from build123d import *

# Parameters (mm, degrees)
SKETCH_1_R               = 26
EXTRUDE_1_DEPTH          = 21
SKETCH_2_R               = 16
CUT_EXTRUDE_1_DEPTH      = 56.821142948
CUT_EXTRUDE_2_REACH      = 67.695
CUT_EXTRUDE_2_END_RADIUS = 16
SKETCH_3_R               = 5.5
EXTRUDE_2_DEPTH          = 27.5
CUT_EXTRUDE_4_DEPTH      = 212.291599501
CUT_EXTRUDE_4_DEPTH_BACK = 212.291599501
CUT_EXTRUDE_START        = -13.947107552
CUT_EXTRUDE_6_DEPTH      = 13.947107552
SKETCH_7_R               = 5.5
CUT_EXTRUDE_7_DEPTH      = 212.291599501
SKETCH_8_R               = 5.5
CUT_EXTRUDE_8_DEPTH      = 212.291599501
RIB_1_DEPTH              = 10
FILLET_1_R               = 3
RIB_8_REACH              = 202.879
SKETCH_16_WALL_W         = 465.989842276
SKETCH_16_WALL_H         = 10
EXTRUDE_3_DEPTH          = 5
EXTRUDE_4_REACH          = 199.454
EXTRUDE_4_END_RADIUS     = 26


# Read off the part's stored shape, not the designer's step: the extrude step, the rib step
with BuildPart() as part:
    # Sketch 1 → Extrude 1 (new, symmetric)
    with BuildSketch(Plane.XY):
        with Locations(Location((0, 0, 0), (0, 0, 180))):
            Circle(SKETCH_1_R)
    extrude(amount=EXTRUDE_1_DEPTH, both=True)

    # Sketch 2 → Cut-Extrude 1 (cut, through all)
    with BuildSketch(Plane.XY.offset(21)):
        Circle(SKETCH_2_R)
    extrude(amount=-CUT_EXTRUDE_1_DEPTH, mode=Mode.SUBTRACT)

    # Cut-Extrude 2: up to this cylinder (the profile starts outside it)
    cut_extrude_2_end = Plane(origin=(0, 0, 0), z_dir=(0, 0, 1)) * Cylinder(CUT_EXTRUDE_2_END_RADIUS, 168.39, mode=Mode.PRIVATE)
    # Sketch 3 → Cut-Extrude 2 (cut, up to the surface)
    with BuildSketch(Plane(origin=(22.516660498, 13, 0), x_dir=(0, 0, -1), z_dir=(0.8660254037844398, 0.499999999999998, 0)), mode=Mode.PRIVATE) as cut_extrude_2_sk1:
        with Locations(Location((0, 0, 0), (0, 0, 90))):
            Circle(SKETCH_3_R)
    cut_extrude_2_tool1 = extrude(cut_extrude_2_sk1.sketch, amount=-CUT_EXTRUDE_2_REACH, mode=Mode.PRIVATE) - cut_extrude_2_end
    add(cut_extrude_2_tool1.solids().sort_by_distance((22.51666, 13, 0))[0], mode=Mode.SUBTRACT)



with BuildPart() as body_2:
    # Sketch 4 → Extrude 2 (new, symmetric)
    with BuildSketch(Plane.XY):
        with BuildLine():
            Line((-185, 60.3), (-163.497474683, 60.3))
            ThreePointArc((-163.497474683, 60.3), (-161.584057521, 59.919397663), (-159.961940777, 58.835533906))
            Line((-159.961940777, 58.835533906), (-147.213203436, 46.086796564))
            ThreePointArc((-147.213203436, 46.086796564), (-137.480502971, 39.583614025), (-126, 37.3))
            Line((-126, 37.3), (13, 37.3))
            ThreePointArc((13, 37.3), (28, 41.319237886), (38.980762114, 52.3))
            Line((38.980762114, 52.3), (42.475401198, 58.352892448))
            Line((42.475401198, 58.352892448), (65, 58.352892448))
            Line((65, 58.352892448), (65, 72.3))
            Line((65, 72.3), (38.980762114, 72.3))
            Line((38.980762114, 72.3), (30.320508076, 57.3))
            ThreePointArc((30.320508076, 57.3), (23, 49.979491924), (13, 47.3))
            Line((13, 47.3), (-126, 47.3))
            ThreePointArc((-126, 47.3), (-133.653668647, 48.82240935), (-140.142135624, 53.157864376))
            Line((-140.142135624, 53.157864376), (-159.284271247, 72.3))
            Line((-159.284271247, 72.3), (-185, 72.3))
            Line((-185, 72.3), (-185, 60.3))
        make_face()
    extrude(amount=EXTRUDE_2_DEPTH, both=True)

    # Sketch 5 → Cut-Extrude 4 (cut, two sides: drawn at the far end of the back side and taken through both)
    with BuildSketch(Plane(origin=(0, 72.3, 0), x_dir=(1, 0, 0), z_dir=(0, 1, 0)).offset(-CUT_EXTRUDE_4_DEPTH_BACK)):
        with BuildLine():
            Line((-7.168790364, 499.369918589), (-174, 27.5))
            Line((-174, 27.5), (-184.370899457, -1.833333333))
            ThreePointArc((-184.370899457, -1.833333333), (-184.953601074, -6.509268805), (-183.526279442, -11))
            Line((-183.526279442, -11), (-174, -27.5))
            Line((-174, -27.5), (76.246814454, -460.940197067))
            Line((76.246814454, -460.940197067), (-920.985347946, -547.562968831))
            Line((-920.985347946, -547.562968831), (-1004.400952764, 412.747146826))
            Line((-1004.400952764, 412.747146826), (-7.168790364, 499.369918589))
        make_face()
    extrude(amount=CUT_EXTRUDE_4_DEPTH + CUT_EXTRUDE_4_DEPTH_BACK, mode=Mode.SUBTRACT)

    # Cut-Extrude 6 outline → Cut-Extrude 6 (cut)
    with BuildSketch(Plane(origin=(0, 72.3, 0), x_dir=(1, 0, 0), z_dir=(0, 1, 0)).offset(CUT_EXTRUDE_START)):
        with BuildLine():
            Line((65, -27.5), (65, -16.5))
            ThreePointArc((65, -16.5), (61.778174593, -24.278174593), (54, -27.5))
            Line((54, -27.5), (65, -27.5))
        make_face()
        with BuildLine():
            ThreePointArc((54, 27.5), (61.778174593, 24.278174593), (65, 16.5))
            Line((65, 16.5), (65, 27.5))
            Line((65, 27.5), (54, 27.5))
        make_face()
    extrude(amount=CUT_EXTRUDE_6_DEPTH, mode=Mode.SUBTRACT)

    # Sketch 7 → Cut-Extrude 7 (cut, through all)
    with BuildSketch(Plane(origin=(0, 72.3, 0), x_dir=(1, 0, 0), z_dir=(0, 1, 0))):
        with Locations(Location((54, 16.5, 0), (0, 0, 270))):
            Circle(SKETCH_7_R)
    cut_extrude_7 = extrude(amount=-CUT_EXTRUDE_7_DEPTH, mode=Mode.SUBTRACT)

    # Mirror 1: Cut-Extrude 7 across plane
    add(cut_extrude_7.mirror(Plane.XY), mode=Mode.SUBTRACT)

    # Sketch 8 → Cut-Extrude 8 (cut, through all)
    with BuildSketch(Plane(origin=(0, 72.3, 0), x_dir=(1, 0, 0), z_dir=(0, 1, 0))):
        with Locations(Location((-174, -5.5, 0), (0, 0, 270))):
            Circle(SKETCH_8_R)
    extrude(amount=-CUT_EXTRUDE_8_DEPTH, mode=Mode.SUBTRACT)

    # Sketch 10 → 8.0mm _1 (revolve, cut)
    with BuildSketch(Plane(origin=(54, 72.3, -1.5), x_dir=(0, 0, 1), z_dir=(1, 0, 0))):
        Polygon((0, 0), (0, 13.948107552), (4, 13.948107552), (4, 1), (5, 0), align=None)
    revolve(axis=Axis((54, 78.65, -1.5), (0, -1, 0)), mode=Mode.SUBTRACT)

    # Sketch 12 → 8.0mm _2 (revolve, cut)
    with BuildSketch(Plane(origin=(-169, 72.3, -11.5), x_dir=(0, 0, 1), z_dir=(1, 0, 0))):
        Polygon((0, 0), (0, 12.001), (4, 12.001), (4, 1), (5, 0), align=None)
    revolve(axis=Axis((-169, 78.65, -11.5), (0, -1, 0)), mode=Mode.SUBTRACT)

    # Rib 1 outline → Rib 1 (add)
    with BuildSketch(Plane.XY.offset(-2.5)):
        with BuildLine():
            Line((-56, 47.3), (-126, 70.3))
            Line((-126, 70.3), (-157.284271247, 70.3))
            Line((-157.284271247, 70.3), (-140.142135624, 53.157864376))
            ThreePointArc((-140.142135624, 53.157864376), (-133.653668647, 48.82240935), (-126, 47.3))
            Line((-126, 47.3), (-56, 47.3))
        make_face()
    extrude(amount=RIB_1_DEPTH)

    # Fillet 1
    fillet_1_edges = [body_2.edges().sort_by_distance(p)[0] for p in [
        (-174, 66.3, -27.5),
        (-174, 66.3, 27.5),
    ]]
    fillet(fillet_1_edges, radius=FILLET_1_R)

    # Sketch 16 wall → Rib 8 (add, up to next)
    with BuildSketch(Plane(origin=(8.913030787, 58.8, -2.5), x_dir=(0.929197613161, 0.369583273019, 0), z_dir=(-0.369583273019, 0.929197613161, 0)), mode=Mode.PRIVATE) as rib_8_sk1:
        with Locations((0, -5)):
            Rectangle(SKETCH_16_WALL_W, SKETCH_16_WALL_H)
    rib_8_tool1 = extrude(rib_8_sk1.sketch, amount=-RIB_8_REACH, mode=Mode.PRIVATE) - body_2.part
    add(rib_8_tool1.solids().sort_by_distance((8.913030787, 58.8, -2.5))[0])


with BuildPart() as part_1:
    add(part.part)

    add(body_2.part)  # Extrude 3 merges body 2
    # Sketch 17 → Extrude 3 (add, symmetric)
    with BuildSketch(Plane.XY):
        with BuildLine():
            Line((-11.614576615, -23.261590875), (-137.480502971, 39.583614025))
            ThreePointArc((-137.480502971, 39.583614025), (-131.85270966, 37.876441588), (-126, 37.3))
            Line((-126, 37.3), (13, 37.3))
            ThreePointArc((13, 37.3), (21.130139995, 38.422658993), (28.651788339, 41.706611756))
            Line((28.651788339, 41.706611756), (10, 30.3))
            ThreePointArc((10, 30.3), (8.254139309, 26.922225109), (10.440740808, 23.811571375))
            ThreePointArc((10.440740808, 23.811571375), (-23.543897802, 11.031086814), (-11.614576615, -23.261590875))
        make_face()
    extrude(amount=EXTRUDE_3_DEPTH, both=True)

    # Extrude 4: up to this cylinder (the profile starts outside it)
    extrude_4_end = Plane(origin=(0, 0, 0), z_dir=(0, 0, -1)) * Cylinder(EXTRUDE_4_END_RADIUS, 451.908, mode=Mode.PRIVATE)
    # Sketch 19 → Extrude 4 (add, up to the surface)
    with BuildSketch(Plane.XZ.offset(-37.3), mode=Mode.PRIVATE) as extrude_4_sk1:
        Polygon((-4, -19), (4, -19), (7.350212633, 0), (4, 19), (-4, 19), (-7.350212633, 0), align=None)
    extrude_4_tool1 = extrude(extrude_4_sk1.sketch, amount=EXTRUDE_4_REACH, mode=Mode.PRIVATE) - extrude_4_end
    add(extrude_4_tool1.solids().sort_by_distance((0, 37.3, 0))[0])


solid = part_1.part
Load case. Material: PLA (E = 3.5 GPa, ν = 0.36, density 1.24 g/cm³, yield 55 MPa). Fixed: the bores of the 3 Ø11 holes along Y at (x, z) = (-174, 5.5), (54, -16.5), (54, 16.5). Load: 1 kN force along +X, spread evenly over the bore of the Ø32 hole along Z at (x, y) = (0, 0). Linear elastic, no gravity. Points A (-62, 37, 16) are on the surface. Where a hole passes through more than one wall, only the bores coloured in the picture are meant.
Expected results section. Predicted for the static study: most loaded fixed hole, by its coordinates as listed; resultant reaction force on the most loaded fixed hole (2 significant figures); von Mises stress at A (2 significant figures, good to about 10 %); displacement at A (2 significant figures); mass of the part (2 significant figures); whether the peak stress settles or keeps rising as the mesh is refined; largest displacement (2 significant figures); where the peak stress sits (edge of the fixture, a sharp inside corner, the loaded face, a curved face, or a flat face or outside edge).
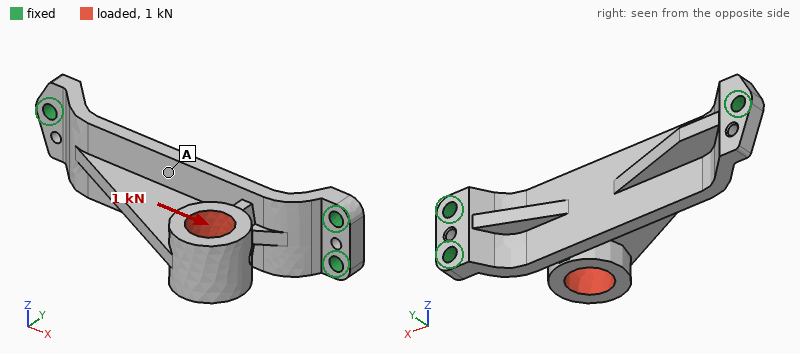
(-174, 5.5)
700 N
0.84 MPa
0.076 mm
320 g
keeps rising
0.18 mm
edge of the fixture
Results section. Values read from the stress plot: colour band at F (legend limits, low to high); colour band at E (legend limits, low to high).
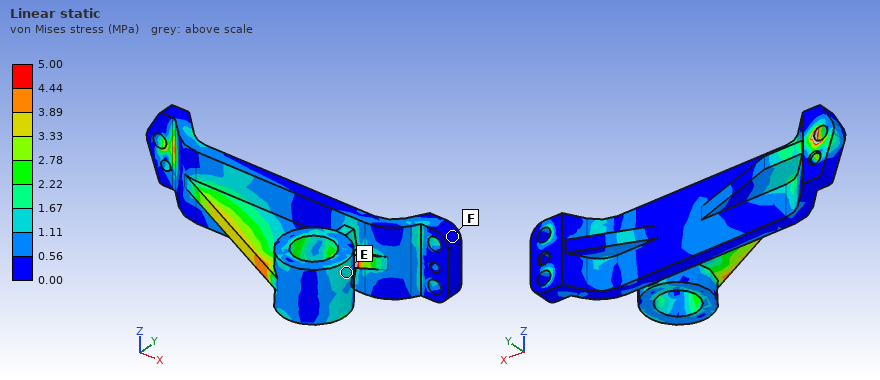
0.00 to 0.56 MPa
1.11 to 1.67 MPa
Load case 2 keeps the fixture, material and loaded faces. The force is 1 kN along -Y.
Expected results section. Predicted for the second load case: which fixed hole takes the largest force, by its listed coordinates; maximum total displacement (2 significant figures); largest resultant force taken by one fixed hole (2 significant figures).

(-174, 5.5)
0.25 mm
700 N
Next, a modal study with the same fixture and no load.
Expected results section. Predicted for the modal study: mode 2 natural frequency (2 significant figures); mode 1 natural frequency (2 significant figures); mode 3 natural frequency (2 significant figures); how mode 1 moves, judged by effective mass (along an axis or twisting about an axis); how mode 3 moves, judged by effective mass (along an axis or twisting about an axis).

760 Hz
440 Hz
920 Hz
along Z
along Y
